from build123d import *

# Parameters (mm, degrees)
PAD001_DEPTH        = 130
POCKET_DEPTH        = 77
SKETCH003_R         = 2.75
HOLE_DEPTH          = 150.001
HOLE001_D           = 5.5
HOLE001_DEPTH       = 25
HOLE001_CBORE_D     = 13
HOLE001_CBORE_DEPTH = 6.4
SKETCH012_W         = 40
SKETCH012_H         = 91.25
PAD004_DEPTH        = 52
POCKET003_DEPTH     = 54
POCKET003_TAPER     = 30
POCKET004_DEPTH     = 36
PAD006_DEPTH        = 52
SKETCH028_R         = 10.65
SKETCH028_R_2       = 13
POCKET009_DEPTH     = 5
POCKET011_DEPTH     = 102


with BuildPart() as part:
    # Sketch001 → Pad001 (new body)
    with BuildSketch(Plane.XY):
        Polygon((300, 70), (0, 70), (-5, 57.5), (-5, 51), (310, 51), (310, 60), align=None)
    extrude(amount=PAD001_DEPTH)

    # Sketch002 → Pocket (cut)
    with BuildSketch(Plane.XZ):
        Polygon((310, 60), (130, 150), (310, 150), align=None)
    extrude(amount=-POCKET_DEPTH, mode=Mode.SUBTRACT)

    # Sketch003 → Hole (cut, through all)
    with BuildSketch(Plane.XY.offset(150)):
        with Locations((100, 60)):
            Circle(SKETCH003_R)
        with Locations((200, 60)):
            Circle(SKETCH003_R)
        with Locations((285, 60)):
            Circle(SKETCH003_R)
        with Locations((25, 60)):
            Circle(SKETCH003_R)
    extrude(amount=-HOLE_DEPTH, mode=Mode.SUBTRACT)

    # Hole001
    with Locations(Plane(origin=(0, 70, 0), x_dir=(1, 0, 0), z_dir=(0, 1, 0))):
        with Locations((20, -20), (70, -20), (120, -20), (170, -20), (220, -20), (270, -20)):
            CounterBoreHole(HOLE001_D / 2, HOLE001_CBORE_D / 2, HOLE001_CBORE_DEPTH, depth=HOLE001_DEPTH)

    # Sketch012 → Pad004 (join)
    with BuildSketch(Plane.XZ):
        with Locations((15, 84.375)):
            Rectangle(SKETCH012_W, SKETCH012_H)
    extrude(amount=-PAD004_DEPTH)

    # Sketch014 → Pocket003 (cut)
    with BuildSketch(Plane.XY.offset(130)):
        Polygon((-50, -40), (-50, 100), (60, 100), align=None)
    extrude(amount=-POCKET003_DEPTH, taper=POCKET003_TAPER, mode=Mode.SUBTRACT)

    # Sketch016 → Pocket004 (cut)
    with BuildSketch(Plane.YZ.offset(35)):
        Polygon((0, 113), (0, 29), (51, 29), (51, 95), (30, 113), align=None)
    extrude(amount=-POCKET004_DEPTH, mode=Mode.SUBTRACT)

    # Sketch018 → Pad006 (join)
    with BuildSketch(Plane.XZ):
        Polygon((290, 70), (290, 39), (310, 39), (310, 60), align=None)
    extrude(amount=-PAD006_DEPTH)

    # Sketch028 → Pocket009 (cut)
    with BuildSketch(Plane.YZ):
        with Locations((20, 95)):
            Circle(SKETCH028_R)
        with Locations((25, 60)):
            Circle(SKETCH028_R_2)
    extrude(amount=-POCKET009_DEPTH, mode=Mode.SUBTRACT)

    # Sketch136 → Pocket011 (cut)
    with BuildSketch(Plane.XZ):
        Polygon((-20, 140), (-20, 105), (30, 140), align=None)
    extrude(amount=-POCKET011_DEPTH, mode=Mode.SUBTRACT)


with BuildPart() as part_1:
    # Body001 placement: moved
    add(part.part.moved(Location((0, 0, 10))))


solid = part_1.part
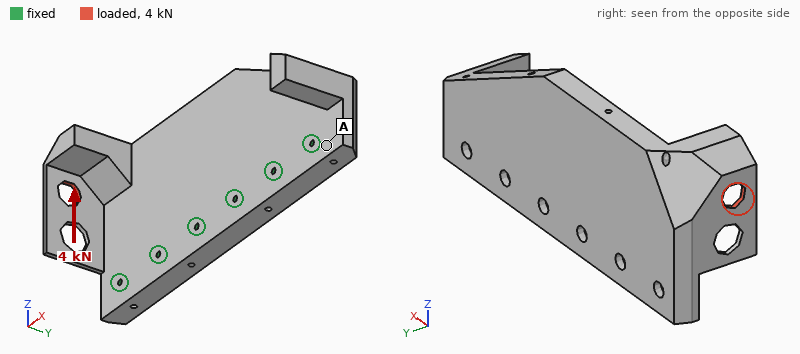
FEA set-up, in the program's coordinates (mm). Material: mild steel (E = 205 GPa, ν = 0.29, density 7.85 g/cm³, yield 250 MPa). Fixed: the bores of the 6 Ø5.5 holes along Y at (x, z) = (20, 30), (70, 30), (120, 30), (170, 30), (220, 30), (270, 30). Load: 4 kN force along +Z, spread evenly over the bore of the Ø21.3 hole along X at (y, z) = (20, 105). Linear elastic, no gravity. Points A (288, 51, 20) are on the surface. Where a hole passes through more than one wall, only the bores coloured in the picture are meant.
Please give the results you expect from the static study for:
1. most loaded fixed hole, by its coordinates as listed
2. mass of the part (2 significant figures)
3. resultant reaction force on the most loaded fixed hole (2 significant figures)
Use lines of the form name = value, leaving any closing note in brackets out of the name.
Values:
most loaded fixed hole, by its coordinates as listed = (20, 30)
mass of the part = 5.6 kg
resultant reaction force on the most loaded fixed hole = 3.7 kN
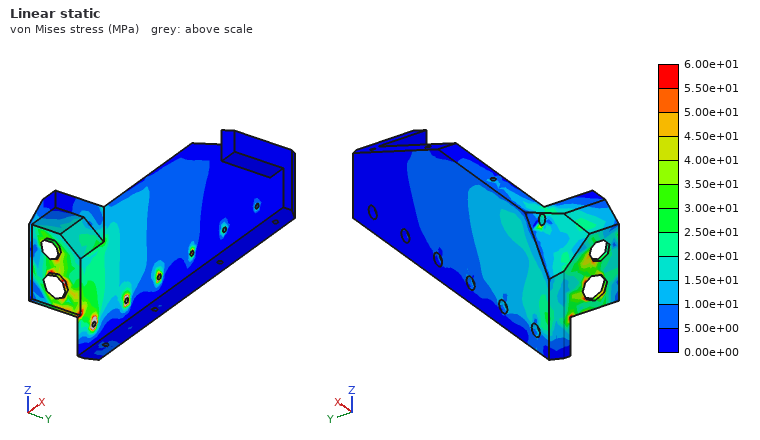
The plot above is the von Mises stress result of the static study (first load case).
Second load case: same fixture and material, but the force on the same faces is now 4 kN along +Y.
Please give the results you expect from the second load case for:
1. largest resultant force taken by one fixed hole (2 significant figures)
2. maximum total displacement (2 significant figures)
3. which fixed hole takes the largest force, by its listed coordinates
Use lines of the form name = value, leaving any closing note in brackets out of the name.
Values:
largest resultant force taken by one fixed hole = 4.3 kN
maximum total displacement = 0.18 mm
which fixed hole takes the largest force, by its listed coordinates = (20, 30)
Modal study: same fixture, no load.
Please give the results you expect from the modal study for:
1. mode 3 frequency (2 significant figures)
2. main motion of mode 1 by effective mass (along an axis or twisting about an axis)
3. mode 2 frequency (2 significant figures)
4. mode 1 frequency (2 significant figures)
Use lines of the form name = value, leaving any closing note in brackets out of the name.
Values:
mode 3 frequency = 1700 Hz
main motion of mode 1 by effective mass = along Y
mode 2 frequency = 1500 Hz
mode 1 frequency = 860 Hz
